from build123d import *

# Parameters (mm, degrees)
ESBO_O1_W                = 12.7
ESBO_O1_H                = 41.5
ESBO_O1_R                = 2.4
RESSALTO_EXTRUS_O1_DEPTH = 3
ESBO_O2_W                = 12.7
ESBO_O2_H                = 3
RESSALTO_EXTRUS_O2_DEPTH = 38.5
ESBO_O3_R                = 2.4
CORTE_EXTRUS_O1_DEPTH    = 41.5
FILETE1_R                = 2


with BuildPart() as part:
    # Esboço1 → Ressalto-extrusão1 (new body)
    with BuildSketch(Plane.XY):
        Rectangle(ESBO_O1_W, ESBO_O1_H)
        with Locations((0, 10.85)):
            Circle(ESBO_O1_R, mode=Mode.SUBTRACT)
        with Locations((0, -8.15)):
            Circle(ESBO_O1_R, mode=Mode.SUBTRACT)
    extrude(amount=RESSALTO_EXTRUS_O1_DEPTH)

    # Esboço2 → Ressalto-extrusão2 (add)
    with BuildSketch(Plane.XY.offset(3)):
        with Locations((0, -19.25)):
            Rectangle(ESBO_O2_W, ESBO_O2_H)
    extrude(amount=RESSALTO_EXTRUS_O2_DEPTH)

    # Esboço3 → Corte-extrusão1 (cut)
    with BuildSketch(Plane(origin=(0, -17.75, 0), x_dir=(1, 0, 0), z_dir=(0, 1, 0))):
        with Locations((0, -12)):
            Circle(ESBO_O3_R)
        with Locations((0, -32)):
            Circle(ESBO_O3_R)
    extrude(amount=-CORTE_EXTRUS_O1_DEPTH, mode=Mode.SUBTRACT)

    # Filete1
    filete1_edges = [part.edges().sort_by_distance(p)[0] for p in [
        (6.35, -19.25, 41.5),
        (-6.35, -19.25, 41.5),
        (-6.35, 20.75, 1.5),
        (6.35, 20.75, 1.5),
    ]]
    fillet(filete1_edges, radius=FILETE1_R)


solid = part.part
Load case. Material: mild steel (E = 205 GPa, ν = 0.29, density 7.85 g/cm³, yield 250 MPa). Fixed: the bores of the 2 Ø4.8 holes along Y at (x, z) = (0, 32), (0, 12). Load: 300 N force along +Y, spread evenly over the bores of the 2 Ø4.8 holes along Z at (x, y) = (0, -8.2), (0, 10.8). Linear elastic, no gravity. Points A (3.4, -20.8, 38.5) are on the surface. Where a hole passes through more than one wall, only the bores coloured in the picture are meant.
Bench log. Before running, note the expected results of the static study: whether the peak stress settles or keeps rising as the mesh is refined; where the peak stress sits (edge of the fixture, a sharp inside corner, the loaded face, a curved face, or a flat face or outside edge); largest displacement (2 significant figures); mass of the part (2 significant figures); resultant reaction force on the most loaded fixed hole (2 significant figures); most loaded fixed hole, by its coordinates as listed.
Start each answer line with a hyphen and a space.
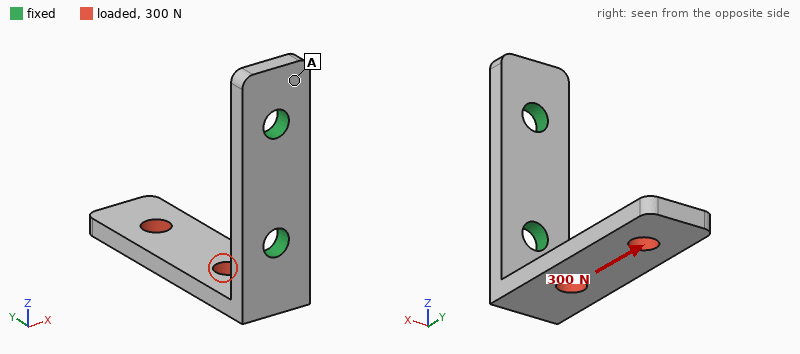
- keeps rising
- edge of the fixture
- 86 µm
- 22 g
- 310 N
- (0, 12)
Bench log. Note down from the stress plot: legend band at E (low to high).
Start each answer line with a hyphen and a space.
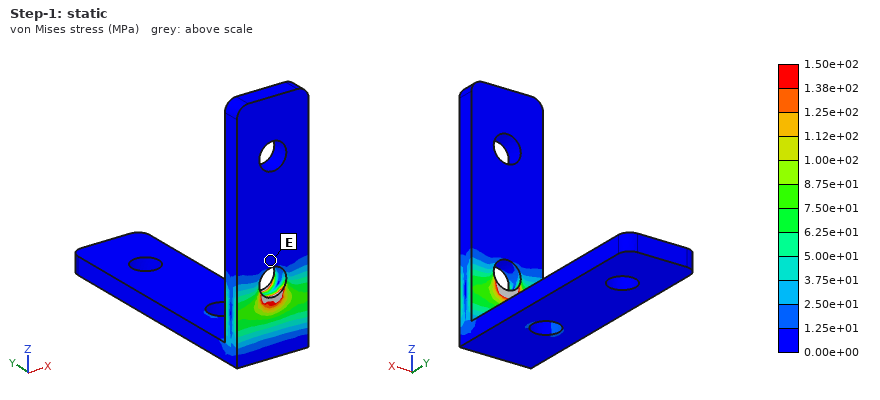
- 0.00e+00 to 1.25e+01 MPa
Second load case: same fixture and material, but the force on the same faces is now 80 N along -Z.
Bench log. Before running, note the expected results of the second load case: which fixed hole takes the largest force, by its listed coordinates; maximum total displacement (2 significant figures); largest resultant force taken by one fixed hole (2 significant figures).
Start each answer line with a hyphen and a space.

- (0, 12)
- 0.21 mm
- 76 N
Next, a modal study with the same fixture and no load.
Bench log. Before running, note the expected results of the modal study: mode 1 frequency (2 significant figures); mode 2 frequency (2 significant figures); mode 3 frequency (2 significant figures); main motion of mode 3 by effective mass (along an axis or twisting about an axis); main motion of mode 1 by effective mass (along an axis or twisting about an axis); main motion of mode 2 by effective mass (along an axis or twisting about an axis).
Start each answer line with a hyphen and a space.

- 1200 Hz
- 2100 Hz
- 6500 Hz
- along Y
- along Z
- along X
